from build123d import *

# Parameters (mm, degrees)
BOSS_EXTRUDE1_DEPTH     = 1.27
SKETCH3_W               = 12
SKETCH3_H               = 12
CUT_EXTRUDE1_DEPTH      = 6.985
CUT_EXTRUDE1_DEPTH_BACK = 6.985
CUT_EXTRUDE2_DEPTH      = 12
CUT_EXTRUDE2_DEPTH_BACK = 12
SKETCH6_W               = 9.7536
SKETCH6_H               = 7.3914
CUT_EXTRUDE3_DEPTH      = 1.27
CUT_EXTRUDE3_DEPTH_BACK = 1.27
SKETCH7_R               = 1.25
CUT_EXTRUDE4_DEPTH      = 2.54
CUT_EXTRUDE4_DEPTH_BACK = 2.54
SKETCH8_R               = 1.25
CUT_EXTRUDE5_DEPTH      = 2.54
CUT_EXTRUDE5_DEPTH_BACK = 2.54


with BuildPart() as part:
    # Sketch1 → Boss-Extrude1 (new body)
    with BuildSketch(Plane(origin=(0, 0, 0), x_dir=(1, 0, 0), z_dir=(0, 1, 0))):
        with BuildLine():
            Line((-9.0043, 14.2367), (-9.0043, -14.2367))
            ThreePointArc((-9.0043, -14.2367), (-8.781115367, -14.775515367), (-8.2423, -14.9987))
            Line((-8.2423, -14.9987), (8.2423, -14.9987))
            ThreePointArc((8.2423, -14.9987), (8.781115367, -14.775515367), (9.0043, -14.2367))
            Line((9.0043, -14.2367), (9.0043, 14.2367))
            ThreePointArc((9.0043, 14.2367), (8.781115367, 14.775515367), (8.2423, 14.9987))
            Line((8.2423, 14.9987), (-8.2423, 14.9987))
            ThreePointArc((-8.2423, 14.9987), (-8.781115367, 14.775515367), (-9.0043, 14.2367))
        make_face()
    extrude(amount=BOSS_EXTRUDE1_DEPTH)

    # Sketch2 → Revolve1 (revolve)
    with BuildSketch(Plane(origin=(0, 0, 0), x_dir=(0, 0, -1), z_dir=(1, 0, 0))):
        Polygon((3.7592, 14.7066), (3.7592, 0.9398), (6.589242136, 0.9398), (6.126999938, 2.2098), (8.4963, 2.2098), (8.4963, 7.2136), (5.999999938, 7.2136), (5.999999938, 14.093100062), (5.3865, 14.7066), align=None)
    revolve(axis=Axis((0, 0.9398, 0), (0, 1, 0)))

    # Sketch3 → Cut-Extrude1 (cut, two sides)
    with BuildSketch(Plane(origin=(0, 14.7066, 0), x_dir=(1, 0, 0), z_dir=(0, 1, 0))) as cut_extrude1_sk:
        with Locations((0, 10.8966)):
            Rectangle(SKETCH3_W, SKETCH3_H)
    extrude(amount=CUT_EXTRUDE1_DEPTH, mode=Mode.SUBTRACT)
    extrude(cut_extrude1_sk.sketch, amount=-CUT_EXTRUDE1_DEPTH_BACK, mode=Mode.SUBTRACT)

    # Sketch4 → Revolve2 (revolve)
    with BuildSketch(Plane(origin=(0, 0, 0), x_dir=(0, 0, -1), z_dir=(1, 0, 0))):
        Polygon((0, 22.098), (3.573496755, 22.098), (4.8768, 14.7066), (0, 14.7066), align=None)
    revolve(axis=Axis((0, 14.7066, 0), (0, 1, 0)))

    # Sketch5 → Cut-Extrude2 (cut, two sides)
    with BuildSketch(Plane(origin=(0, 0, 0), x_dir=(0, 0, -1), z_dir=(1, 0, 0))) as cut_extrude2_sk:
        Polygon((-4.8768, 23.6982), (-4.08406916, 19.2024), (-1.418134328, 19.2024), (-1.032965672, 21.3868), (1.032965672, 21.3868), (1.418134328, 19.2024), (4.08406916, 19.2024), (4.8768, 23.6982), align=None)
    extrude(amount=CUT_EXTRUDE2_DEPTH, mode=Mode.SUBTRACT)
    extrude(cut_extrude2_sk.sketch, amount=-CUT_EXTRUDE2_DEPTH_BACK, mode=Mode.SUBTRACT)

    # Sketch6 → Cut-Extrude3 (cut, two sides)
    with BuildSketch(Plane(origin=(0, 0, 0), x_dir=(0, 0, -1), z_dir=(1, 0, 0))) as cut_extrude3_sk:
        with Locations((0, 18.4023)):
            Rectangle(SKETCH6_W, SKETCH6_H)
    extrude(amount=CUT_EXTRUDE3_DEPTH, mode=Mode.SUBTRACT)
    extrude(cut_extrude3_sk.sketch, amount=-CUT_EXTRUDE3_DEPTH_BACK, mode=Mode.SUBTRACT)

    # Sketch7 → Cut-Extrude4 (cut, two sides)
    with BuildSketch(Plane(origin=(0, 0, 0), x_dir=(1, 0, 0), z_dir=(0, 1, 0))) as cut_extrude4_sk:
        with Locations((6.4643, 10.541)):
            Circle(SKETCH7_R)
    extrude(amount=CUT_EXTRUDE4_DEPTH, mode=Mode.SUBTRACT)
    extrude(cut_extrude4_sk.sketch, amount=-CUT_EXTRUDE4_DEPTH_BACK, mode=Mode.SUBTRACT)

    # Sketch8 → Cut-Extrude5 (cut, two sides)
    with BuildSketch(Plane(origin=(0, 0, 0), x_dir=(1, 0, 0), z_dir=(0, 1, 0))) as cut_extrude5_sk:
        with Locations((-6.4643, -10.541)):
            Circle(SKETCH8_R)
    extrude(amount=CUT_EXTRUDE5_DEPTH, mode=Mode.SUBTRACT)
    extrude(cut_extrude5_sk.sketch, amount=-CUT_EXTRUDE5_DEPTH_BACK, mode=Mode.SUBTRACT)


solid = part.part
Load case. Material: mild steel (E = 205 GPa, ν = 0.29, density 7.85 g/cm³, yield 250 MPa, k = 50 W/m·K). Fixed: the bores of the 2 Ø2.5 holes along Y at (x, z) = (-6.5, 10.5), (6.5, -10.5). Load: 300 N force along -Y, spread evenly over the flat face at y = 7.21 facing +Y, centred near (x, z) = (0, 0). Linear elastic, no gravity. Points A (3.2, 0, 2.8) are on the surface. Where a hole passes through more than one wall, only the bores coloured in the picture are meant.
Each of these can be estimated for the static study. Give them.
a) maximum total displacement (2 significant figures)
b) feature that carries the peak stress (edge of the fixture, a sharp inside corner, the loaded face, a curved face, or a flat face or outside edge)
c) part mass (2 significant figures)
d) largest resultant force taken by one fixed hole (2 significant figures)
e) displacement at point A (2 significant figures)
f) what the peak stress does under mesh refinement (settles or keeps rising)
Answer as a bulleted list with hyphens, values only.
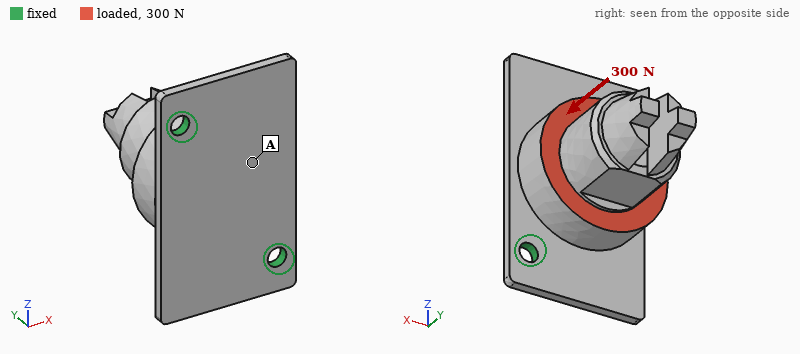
- 12 µm
- edge of the fixture
- 18 g
- 160 N
- 11 µm
- keeps rising
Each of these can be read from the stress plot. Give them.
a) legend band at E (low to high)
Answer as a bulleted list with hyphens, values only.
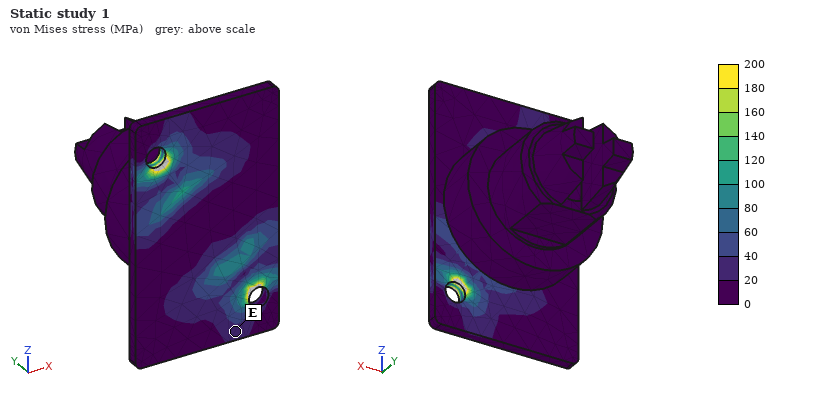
- 20 to 40 MPa
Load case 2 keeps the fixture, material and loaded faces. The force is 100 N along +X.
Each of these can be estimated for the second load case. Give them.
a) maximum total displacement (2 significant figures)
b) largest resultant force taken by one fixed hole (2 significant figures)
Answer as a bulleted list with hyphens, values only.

- 47 µm
- 53 N
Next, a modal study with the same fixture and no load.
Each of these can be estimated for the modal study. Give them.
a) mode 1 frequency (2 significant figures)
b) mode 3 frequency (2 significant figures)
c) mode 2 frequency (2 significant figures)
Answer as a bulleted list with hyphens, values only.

- 2200 Hz
- 6700 Hz
- 6400 Hz
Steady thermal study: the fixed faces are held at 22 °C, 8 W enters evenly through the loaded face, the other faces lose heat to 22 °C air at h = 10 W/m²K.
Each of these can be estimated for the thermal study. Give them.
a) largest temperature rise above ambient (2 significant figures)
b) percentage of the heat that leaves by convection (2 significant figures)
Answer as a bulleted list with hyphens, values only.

- 46 K
- 10 %
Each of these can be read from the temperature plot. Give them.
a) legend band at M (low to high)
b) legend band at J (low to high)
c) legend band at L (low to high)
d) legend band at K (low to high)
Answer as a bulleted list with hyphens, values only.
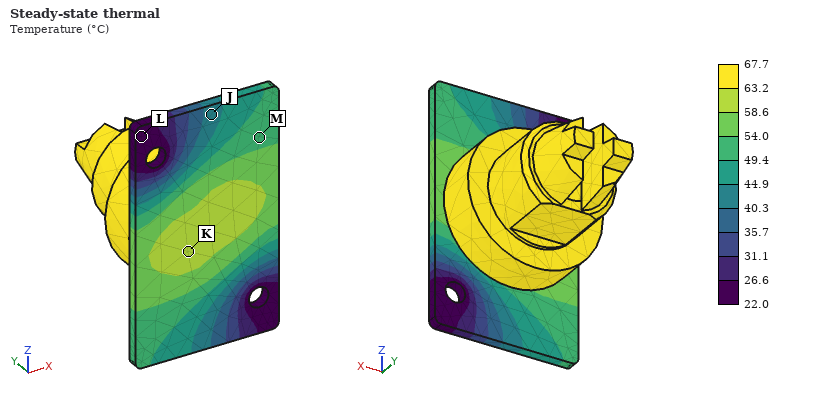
- 49.4 to 54.0 °C
- 40.3 to 44.9 °C
- 22.0 to 26.6 °C
- 58.6 to 63.2 °C
